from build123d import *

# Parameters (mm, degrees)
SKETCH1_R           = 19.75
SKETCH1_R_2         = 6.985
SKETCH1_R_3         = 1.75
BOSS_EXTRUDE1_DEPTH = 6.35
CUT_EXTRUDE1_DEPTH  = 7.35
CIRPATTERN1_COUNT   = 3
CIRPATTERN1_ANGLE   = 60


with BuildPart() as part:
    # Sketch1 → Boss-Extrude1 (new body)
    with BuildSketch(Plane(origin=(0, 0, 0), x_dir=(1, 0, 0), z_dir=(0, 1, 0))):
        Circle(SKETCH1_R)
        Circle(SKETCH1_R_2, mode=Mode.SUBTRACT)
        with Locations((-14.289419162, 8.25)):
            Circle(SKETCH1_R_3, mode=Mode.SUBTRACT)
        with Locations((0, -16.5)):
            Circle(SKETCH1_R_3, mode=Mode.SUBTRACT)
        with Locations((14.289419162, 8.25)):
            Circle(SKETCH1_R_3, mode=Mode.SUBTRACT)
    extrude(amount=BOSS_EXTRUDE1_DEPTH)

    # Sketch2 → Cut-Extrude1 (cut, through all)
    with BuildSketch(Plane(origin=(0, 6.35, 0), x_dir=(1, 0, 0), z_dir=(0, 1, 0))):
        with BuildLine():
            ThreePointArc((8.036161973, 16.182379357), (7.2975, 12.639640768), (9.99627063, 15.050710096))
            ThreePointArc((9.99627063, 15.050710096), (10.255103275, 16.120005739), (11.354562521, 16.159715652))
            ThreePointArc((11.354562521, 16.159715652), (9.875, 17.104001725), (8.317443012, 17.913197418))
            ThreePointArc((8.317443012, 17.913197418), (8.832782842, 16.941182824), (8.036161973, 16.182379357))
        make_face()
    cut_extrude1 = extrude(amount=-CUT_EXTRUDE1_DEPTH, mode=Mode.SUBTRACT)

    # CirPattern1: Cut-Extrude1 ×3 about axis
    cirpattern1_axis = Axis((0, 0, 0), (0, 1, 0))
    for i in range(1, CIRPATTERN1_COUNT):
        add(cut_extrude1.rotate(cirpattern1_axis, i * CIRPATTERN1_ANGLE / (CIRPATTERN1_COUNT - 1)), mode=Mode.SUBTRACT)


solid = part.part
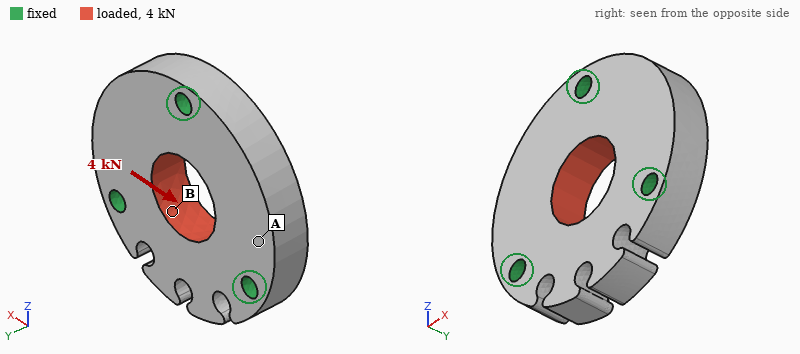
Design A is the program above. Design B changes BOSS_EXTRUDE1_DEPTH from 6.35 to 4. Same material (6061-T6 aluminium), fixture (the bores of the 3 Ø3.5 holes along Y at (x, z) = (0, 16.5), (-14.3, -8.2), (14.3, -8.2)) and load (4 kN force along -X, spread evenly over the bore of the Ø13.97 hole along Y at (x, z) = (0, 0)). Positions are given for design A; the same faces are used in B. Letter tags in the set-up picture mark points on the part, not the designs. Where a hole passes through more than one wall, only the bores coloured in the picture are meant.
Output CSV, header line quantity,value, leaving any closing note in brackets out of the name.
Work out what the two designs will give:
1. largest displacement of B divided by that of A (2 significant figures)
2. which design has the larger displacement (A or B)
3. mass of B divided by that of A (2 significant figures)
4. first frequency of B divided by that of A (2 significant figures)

quantity,value
largest displacement of B divided by that of A,1.6
which design has the larger displacement,B
mass of B divided by that of A,0.63
first frequency of B divided by that of A,0.74
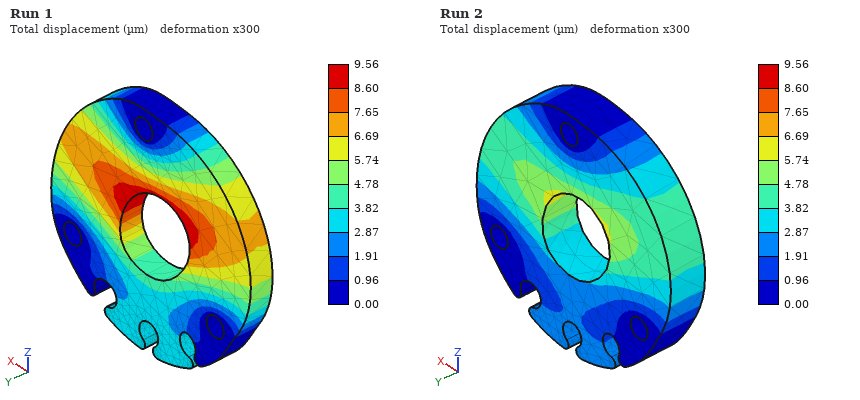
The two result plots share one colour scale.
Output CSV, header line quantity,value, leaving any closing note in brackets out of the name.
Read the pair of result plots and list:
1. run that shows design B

quantity,value
run that shows design B,Run 1
